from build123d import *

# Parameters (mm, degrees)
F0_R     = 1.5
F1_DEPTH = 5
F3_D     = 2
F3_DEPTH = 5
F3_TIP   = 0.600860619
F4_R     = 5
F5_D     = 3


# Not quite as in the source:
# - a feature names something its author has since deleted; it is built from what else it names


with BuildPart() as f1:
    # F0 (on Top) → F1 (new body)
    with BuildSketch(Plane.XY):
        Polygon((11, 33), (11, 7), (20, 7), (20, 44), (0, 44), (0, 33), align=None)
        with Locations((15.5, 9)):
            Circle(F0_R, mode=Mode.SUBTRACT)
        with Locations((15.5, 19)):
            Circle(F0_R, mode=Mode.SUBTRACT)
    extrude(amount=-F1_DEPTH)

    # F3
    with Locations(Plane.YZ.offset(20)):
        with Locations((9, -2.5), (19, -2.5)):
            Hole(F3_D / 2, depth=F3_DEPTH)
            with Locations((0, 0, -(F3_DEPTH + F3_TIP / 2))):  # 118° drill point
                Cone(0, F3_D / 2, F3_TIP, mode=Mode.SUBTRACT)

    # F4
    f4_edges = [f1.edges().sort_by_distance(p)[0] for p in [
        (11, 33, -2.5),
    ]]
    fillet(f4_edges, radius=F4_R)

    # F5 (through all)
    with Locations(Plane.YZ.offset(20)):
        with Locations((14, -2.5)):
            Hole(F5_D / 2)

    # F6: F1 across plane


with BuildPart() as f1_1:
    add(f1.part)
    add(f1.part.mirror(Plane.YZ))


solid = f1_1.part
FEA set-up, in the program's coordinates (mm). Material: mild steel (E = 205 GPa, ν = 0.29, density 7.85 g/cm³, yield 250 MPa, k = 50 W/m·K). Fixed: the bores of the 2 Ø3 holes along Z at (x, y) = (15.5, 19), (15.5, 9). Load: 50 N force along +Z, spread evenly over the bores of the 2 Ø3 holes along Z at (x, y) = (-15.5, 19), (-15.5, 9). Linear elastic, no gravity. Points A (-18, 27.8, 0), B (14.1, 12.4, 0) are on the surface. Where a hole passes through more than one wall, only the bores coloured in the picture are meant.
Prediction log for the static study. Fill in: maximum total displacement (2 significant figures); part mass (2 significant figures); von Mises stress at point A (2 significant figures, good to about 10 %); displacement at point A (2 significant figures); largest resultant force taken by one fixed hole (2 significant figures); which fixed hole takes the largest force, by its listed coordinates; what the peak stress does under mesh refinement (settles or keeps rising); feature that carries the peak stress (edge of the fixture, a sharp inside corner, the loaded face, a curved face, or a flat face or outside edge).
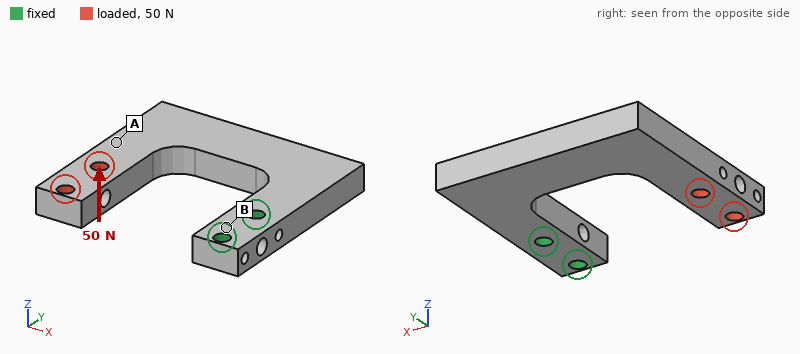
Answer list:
0.12 mm
34 g
17 MPa
0.069 mm
48 N
(15.5, 19)
keeps rising
edge of the fixture
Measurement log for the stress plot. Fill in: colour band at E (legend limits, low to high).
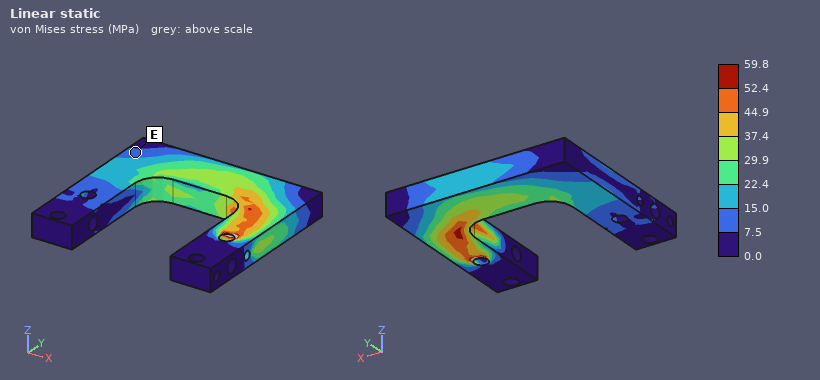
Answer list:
7.5 to 15.0 MPa
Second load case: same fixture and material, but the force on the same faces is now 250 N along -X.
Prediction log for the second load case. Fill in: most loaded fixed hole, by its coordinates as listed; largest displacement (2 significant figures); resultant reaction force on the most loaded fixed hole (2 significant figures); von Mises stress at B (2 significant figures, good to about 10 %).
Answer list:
(15.5, 19)
99 µm
200 N
5.7 MPa
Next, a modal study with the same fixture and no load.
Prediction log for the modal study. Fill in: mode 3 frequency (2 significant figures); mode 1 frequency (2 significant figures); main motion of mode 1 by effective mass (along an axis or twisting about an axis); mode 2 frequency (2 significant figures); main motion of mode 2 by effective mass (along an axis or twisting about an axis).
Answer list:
2500 Hz
1200 Hz
along Z
2000 Hz
along Y
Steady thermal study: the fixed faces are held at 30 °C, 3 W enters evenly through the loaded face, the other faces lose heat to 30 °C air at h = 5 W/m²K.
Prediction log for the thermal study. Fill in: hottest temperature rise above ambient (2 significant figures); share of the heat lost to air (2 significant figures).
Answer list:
75 K
16 %
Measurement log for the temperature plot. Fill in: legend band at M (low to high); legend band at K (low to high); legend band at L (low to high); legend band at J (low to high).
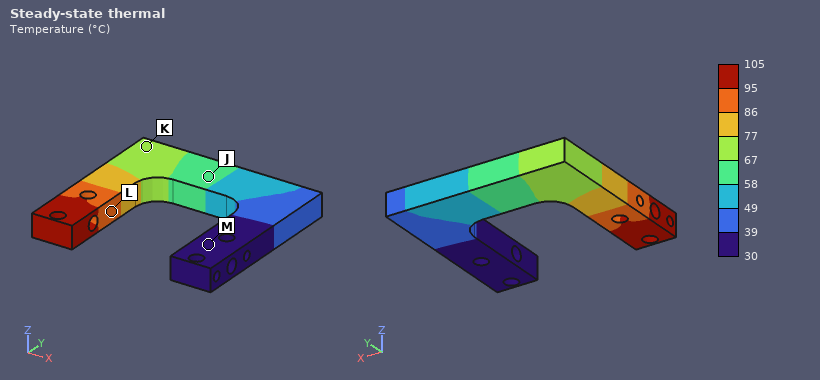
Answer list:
30 to 39 °C
67 to 77 °C
86 to 95 °C
58 to 67 °C
